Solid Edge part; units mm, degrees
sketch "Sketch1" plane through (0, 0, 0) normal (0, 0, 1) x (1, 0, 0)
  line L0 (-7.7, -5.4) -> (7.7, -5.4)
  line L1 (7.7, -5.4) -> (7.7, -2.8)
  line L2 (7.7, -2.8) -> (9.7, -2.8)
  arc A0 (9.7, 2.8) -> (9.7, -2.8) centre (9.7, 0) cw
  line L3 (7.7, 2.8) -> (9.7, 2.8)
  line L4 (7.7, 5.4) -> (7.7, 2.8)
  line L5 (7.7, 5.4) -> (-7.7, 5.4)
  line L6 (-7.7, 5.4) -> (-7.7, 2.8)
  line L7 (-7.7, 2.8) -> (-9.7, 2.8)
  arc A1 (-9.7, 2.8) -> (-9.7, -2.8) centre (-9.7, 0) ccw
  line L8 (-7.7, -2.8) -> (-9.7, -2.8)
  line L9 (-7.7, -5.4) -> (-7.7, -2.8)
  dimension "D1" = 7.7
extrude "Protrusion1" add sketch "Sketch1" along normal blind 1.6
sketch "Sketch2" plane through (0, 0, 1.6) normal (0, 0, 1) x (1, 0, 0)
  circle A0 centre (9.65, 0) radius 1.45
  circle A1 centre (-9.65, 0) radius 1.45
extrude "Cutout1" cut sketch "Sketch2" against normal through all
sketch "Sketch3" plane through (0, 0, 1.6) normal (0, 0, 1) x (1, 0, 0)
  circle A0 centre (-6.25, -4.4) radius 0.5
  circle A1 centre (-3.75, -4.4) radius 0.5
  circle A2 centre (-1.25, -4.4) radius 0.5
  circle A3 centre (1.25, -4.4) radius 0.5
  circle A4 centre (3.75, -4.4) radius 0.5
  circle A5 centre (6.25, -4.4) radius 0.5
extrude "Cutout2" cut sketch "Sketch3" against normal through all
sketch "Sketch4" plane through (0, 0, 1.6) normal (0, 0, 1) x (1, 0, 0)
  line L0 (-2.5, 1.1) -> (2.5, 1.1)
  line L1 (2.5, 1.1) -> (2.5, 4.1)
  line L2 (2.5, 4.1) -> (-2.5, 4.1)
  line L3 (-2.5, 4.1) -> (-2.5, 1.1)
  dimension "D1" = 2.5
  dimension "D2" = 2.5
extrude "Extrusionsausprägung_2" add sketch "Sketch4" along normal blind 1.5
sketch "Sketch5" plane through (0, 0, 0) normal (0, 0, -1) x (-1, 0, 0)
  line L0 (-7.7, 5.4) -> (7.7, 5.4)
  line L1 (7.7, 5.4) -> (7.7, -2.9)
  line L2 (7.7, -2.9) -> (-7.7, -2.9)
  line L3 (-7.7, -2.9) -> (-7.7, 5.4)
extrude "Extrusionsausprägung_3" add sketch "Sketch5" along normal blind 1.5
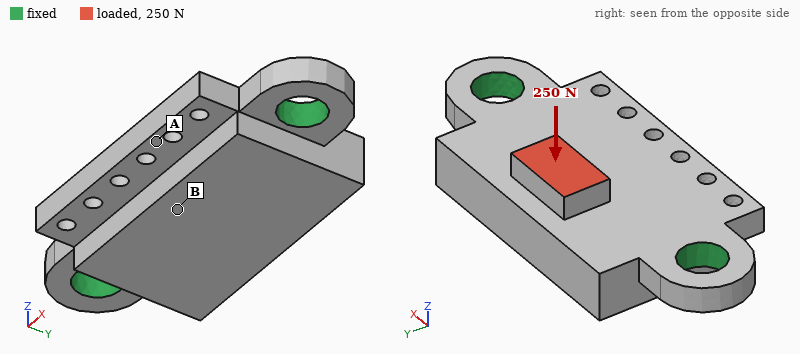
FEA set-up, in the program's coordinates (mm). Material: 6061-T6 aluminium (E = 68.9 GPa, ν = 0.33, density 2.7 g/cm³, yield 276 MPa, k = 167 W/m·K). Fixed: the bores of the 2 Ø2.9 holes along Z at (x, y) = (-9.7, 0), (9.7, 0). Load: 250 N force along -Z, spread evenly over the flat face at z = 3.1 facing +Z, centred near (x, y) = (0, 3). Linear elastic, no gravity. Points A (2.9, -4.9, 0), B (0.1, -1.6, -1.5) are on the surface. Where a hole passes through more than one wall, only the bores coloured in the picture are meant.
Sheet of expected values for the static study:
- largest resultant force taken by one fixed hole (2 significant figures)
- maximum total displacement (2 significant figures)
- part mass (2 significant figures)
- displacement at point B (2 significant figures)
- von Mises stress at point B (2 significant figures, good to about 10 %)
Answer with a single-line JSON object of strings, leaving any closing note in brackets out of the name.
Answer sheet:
{"largest resultant force taken by one fixed hole": "170 N", "maximum total displacement": "23 µm", "part mass": "1.4 g", "displacement at point B": "7.1 µm", "von Mises stress at point B": "35 MPa"}
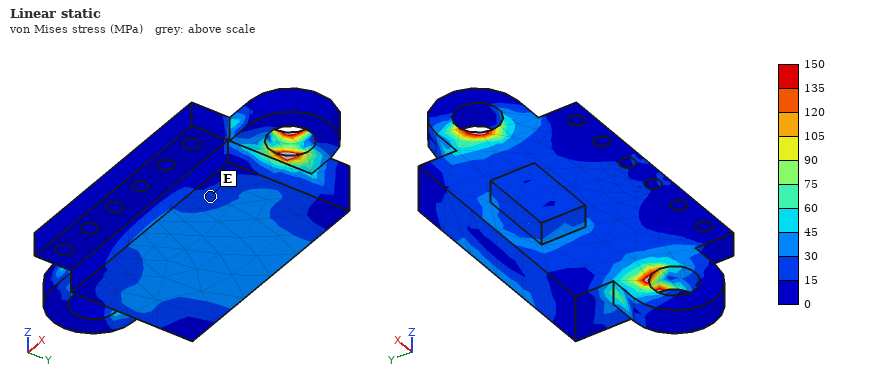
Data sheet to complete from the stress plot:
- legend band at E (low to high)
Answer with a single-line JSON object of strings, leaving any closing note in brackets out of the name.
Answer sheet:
{"legend band at E": "15 to 30 MPa"}
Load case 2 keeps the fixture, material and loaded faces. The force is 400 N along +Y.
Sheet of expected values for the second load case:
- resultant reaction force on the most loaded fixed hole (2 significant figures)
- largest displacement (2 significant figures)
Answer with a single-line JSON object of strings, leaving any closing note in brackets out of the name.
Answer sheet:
{"resultant reaction force on the most loaded fixed hole": "210 N", "largest displacement": "29 µm"}
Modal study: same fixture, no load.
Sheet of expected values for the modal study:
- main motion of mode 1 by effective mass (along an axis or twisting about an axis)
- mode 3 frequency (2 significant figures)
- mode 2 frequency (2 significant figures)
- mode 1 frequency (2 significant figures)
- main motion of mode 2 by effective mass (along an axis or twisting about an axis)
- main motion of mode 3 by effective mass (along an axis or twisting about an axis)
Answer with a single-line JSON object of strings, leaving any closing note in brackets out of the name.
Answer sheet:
{"main motion of mode 1 by effective mass": "along Z", "mode 3 frequency": "49 kHz", "mode 2 frequency": "30 kHz", "mode 1 frequency": "24 kHz", "main motion of mode 2 by effective mass": "along Z", "main motion of mode 3 by effective mass": "along Y"}
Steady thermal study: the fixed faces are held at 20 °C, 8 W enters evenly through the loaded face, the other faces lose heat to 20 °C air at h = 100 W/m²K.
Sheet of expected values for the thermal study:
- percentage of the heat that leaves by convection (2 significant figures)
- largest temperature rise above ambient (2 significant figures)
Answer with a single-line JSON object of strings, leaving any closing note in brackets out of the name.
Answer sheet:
{"percentage of the heat that leaves by convection": "4.6 %", "largest temperature rise above ambient": "17 K"}
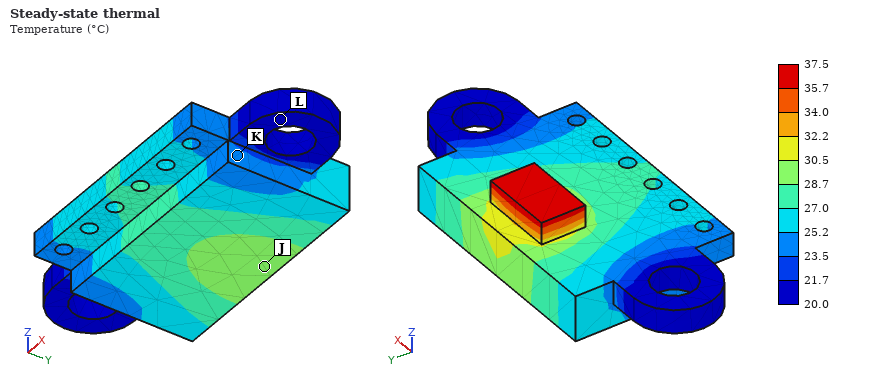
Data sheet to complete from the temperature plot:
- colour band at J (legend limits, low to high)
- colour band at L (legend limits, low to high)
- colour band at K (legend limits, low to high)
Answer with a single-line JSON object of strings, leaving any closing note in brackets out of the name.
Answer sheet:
{"colour band at J": "28.7 to 30.5 °C", "colour band at L": "20.0 to 21.7 °C", "colour band at K": "23.5 to 25.2 °C"}
